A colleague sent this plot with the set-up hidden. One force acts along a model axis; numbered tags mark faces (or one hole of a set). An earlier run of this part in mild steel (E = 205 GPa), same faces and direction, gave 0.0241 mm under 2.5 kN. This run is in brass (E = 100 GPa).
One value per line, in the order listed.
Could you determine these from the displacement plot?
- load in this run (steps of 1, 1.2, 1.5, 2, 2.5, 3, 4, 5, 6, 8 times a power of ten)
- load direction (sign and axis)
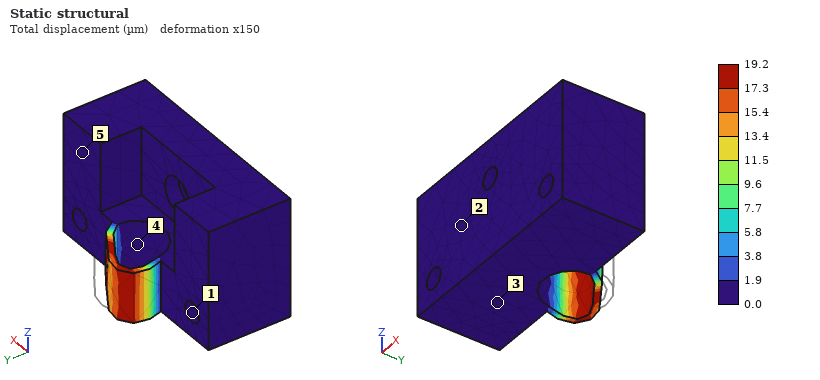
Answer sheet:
1 kN
-X
